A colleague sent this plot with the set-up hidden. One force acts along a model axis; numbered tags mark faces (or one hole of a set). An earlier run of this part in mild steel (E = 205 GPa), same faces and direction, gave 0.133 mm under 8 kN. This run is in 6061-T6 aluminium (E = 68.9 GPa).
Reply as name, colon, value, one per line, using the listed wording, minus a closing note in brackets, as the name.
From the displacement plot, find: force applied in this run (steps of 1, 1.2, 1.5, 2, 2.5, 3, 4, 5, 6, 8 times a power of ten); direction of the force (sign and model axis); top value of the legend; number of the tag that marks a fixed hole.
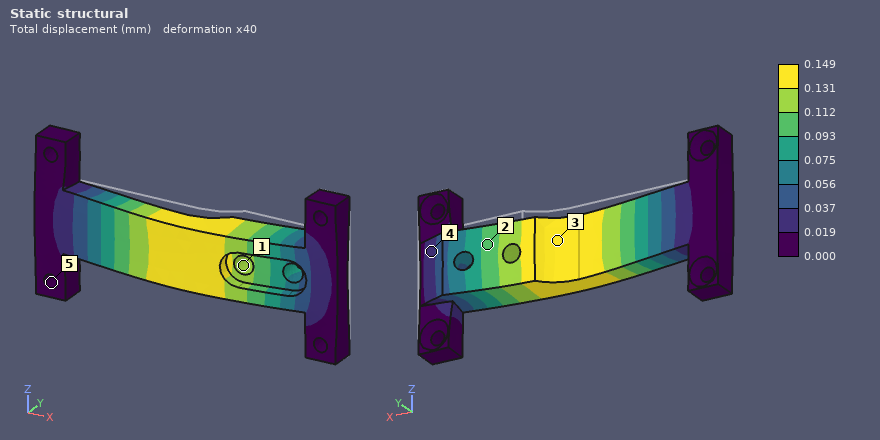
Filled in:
force applied in this run: 3 kN
direction of the force: -Y
top value of the legend: 0.149 mm
number of the tag that marks a fixed hole: 5
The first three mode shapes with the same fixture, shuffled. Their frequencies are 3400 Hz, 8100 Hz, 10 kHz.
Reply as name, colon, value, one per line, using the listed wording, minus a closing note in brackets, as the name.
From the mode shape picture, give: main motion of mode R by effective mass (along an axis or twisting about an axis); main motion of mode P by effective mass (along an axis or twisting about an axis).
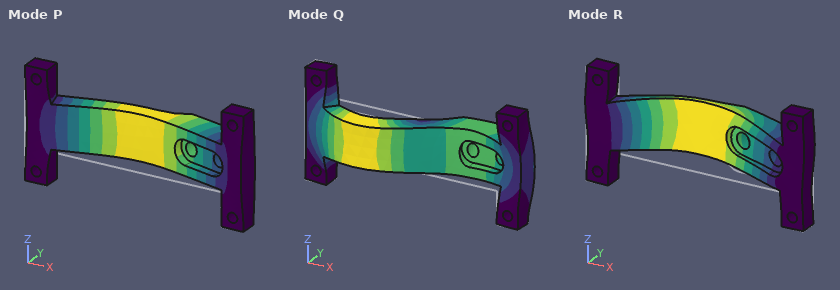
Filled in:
main motion of mode R by effective mass: along Z
main motion of mode P by effective mass: along Y
